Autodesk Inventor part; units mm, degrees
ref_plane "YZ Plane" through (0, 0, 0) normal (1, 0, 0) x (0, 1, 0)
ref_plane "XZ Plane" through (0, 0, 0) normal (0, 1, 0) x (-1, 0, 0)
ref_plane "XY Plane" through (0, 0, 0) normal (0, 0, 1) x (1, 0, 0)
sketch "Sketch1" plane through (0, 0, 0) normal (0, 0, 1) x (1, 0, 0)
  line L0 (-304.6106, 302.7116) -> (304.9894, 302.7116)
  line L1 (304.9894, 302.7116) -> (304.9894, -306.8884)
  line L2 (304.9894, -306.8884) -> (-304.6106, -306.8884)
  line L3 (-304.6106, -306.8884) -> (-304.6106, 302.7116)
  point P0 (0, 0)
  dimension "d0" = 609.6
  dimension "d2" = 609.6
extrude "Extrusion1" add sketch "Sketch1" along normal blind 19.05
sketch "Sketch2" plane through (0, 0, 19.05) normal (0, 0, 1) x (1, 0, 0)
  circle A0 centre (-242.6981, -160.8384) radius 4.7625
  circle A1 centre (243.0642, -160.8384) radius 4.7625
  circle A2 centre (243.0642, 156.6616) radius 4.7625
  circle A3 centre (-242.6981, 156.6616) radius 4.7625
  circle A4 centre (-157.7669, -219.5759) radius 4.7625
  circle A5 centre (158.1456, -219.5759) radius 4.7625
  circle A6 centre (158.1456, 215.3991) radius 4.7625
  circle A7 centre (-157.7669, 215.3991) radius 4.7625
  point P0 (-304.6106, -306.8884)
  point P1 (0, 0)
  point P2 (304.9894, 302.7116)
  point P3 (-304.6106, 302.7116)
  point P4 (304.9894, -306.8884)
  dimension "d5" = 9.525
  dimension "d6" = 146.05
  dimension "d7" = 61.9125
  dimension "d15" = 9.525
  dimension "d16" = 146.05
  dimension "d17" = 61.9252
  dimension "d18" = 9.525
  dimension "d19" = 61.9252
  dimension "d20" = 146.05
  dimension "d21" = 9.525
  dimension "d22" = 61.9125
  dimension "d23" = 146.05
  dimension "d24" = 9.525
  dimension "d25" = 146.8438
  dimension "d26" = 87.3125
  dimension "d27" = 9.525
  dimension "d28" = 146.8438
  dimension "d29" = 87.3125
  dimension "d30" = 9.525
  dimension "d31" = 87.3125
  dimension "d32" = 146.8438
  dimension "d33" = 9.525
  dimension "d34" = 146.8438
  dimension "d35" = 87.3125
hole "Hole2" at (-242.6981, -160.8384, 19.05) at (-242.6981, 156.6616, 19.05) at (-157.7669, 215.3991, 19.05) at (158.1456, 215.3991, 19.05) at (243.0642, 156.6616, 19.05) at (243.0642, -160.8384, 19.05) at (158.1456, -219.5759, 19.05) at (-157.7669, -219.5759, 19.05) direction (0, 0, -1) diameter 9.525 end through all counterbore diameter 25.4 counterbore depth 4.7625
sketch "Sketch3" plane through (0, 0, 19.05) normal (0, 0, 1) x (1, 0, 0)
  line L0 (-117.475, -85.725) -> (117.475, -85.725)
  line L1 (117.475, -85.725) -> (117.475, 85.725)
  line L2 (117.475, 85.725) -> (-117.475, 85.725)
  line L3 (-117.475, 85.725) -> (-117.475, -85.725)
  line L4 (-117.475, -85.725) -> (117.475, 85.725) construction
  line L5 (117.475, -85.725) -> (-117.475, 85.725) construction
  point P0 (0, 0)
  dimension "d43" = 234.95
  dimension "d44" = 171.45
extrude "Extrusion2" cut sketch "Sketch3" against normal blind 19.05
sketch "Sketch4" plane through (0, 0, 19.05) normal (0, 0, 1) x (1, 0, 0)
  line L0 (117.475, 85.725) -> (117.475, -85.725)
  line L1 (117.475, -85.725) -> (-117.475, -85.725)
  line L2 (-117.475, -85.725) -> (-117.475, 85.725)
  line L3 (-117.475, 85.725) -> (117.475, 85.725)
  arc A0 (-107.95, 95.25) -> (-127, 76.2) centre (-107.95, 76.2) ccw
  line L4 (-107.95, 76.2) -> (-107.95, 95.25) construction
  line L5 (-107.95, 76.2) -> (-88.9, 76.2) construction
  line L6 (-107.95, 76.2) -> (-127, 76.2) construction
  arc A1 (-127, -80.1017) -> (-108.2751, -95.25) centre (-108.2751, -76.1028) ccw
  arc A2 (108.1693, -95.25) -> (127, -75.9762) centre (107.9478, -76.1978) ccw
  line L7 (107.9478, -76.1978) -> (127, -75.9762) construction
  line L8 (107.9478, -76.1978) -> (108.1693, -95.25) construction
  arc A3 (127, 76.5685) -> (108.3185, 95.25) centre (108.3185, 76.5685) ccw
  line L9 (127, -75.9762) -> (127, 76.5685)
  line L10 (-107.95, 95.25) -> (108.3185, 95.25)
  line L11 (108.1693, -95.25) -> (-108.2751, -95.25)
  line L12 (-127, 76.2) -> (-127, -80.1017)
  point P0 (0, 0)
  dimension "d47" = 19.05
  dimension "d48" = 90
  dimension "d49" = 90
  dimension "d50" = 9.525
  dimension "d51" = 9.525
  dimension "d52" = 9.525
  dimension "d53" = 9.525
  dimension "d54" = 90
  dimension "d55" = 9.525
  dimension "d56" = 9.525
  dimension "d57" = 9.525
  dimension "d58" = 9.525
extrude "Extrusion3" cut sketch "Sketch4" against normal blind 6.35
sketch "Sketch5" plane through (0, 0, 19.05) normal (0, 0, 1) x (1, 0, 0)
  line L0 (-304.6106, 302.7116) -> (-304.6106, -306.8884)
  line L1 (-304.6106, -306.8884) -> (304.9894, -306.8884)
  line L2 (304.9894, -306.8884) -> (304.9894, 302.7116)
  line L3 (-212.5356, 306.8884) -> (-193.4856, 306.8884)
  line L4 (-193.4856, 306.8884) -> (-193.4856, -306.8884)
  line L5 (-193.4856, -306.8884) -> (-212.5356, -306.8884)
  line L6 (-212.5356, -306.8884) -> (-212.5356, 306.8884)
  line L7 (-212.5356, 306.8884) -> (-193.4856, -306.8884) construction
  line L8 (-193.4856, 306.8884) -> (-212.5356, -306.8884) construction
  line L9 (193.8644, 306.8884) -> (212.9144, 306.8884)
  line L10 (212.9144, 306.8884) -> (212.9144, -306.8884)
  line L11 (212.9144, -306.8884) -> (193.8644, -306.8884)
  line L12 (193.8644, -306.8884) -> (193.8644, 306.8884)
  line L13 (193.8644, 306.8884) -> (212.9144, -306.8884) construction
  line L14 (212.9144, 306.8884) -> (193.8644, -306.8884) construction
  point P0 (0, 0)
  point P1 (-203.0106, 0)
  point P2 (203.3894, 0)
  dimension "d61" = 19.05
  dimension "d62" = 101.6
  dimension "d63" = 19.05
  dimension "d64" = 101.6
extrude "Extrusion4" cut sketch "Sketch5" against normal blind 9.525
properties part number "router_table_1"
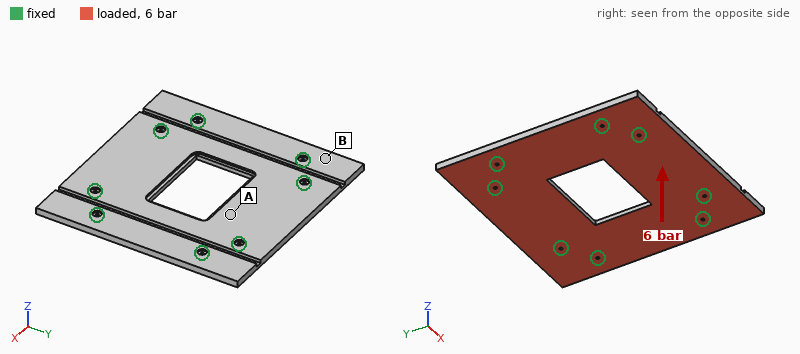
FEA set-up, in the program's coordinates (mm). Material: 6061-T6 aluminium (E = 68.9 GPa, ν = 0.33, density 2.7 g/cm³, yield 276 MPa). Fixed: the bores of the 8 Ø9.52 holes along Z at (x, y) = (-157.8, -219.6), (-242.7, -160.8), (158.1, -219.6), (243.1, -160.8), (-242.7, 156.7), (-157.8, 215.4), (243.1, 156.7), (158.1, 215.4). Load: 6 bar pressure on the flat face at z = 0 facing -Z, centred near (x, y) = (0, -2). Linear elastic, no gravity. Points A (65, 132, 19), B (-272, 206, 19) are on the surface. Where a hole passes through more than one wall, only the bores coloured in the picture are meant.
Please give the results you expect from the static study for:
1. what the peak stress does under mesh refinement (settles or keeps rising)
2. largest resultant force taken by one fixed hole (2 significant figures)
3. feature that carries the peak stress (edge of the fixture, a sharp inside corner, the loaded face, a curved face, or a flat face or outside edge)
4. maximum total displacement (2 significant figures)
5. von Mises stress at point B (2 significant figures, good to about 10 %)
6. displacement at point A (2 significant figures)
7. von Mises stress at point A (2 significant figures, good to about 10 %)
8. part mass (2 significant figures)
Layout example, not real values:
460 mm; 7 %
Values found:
keeps rising; 31 kN; edge of the fixture; 2.0 mm; 22 MPa; 1.3 mm; 52 MPa; 16 kg
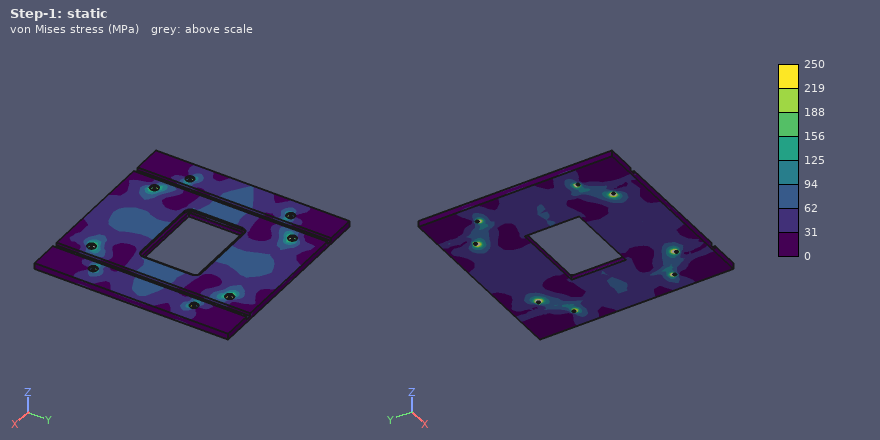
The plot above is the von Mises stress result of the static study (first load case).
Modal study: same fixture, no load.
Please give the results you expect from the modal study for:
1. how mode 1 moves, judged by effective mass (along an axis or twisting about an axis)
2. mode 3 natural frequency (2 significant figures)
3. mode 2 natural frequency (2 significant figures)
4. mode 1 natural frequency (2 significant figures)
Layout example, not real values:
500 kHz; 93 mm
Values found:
along Z; 670 Hz; 660 Hz; 470 Hz
